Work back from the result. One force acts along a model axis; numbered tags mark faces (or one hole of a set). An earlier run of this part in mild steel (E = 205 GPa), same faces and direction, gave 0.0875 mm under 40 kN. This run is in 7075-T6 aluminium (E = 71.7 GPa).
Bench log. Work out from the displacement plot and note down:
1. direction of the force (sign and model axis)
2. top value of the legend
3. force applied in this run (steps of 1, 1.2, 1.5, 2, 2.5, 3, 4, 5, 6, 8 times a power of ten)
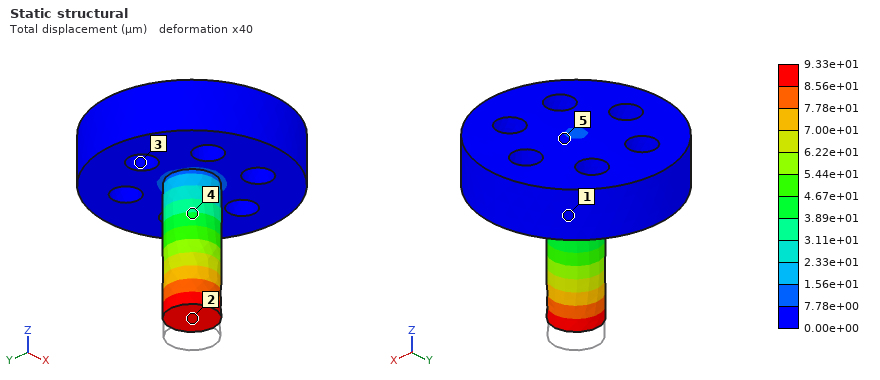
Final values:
+Z
9.33e+01 µm
15 kN
